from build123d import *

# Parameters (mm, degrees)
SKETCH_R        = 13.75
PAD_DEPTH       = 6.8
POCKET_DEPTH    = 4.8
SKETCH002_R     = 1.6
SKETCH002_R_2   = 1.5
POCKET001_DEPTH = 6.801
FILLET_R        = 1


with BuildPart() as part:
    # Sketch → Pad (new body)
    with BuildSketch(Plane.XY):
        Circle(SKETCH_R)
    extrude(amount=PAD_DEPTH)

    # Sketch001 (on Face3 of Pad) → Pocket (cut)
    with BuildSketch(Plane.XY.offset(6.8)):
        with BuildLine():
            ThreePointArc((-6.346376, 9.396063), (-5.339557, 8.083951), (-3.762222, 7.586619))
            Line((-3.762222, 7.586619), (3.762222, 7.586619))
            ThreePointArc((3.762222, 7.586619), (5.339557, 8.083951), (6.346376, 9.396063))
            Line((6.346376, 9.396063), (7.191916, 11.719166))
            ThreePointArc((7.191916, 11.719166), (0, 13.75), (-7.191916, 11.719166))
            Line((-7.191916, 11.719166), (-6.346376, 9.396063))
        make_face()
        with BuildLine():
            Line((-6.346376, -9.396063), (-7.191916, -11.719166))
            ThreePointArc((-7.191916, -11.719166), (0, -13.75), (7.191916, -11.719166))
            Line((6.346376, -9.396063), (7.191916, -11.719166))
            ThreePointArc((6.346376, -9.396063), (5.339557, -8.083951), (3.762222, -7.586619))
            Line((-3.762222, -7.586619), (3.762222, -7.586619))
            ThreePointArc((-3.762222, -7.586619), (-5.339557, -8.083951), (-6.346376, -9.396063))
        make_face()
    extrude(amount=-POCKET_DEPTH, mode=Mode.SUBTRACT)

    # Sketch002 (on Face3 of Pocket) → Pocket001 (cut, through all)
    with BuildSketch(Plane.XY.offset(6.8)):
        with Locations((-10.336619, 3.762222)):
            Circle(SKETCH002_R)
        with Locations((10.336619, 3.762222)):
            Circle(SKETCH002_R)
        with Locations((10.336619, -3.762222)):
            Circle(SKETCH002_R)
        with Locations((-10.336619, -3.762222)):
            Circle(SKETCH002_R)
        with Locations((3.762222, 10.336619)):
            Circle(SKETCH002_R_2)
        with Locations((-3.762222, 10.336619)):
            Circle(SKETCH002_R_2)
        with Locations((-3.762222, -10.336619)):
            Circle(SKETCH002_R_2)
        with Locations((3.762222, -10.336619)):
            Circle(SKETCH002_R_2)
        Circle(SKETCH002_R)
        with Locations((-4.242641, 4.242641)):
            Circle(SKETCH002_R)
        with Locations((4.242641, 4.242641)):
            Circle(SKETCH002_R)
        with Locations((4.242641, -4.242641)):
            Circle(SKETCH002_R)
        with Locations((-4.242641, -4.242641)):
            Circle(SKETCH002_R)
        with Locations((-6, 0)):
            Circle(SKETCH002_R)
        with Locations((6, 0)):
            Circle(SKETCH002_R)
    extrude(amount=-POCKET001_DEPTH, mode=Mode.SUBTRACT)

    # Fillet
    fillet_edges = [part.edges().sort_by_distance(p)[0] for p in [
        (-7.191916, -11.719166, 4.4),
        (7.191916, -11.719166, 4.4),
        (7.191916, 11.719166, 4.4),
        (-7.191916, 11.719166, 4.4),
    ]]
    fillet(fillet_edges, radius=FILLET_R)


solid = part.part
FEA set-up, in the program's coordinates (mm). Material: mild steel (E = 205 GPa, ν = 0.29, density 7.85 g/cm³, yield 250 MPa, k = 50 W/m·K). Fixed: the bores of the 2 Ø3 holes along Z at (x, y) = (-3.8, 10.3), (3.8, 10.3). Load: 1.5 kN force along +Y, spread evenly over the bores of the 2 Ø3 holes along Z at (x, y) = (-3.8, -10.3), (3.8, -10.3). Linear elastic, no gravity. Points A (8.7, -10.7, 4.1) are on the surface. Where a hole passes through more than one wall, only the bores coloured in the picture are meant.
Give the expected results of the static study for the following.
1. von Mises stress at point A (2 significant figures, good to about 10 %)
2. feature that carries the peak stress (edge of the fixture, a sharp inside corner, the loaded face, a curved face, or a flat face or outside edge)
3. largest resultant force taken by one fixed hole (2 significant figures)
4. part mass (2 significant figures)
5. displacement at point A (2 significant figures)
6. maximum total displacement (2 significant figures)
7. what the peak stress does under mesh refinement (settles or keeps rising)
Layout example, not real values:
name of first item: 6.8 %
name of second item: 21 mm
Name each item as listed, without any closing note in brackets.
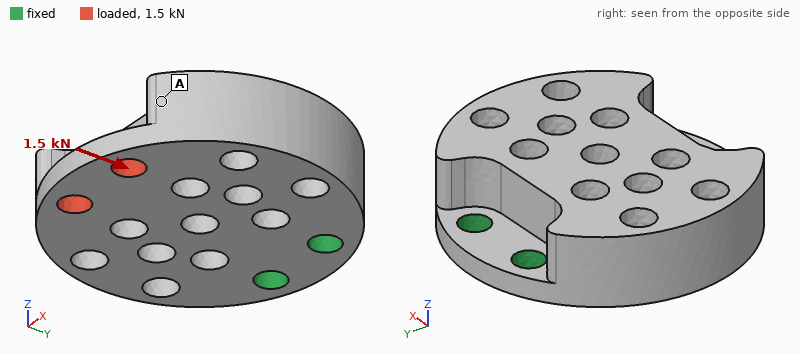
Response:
von Mises stress at point A: 14 MPa
feature that carries the peak stress: a sharp inside corner
largest resultant force taken by one fixed hole: 750 N
part mass: 21 g
displacement at point A: 7.5 µm
maximum total displacement: 13 µm
what the peak stress does under mesh refinement: keeps rising
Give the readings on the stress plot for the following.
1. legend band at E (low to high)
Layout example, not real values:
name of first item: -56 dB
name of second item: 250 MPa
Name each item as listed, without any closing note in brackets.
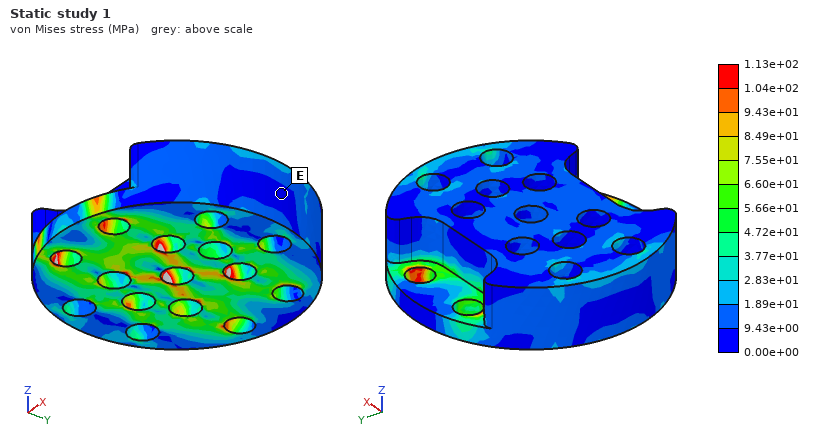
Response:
legend band at E: 0.00e+00 to 9.43e+00 MPa
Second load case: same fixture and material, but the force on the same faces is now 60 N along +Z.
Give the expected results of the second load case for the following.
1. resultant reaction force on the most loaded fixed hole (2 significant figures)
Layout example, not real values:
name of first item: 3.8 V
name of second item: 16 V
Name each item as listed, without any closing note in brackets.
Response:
resultant reaction force on the most loaded fixed hole: 31 N
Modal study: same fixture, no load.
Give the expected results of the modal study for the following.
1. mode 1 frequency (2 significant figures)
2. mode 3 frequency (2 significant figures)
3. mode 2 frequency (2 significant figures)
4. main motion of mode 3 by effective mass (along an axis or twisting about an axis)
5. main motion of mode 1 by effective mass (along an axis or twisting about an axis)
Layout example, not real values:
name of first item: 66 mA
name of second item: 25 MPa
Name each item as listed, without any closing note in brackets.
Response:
mode 1 frequency: 3600 Hz
mode 3 frequency: 11 kHz
mode 2 frequency: 9200 Hz
main motion of mode 3 by effective mass: along X
main motion of mode 1 by effective mass: along Z
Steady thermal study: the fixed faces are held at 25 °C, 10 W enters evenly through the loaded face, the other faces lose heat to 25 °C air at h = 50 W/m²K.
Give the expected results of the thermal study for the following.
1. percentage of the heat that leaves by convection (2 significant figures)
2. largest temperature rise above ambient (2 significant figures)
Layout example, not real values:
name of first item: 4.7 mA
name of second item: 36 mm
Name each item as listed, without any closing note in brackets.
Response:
percentage of the heat that leaves by convection: 28 %
largest temperature rise above ambient: 66 K
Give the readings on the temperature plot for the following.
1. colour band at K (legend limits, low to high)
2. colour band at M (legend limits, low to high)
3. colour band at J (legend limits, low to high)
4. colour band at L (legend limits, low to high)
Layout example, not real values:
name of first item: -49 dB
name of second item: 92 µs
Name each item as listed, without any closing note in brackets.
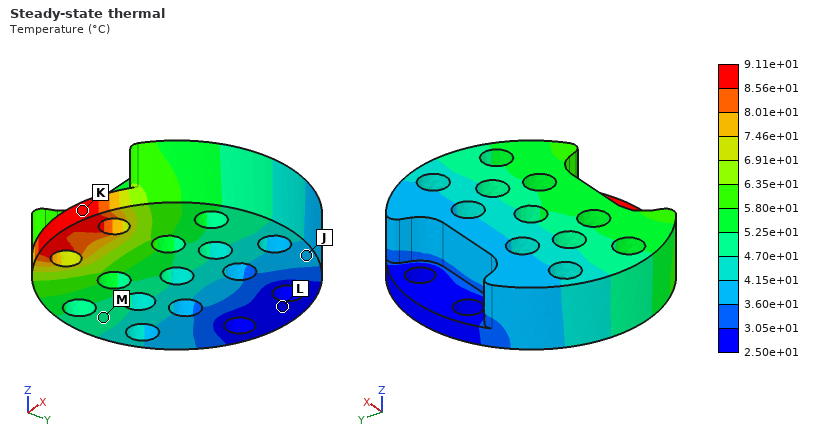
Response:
colour band at K: 8.56e+01 to 9.11e+01 °C
colour band at M: 4.70e+01 to 5.25e+01 °C
colour band at J: 3.60e+01 to 4.15e+01 °C
colour band at L: 2.50e+01 to 3.05e+01 °C
